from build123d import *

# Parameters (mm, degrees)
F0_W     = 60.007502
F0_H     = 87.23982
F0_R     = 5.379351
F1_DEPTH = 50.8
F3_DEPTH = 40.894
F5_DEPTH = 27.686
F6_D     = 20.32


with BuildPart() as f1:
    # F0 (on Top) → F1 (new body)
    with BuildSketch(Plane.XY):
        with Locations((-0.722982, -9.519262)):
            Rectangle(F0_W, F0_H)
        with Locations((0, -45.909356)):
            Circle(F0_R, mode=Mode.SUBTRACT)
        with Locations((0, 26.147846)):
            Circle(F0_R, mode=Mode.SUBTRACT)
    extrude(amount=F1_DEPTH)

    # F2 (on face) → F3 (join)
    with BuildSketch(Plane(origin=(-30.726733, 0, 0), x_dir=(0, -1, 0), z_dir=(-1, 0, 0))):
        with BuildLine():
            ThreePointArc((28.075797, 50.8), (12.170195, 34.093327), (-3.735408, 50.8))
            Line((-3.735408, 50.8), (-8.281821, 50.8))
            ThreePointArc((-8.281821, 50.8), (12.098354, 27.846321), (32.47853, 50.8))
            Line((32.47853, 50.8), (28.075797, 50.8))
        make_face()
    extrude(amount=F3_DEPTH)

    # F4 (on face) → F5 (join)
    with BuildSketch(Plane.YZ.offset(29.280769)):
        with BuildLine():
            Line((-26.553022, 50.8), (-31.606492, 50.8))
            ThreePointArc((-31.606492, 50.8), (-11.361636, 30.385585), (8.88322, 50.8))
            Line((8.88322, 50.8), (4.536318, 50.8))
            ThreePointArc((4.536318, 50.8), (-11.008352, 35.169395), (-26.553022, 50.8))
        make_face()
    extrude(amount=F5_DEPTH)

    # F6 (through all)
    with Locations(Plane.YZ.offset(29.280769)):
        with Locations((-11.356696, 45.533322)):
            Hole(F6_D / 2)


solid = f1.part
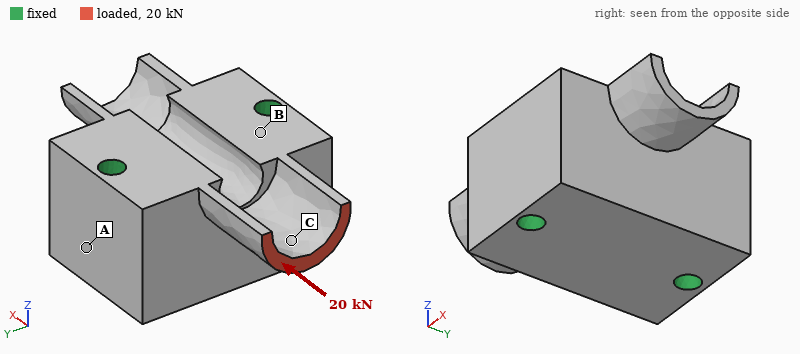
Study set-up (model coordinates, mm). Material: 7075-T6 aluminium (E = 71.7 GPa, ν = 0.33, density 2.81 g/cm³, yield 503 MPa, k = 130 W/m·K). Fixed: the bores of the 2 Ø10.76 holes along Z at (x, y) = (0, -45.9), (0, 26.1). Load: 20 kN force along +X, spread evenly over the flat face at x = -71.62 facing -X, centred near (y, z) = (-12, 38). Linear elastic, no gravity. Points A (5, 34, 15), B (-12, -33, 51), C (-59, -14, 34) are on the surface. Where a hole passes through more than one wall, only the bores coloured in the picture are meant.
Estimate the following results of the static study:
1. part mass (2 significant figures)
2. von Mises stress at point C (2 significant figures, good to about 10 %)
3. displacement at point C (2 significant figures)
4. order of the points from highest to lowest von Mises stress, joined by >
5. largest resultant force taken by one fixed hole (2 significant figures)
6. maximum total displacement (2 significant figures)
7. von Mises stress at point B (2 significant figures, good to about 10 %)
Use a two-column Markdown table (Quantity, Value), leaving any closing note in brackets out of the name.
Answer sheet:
| Quantity | Value |
|---|---|
| part mass | 740 g |
| von Mises stress at point C | 59 MPa |
| displacement at point C | 35 µm |
| order of the points from highest to lowest von Mises stress, joined by > | C > B > A |
| largest resultant force taken by one fixed hole | 11 kN |
| maximum total displacement | 49 µm |
| von Mises stress at point B | 21 MPa |
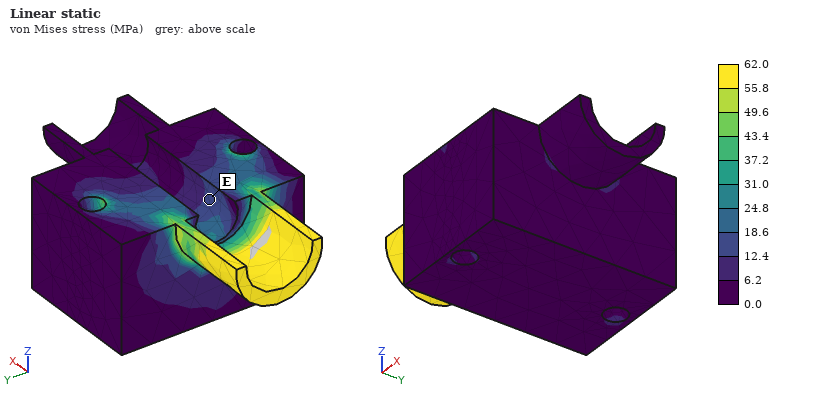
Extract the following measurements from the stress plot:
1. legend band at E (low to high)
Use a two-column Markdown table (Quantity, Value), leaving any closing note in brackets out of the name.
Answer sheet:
| Quantity | Value |
|---|---|
| legend band at E | 12.4 to 18.6 MPa |
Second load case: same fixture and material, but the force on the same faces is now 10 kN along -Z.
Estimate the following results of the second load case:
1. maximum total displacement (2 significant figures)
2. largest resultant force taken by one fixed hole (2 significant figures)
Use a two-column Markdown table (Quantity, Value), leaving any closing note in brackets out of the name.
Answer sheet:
| Quantity | Value |
|---|---|
| maximum total displacement | 0.55 mm |
| largest resultant force taken by one fixed hole | 5.3 kN |
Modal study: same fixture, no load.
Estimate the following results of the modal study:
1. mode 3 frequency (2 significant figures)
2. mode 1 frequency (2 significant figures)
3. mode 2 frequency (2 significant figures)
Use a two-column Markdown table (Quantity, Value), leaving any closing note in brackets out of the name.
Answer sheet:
| Quantity | Value |
|---|---|
| mode 3 frequency | 7800 Hz |
| mode 1 frequency | 5100 Hz |
| mode 2 frequency | 6400 Hz |
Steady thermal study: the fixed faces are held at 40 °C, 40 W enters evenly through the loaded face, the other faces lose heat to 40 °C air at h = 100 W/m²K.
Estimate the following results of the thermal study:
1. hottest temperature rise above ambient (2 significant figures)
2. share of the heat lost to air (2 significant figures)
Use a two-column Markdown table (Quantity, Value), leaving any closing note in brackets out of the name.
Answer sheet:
| Quantity | Value |
|---|---|
| hottest temperature rise above ambient | 36 K |
| share of the heat lost to air | 31 % |
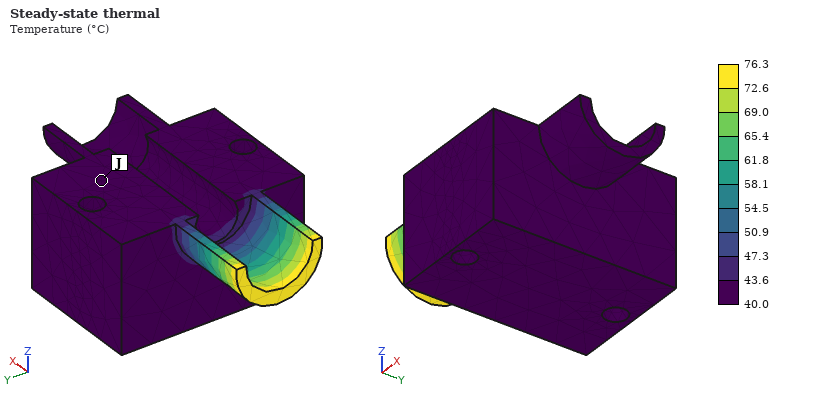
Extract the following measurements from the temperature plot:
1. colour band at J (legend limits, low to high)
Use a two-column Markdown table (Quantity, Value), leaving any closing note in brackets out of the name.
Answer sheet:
| Quantity | Value |
|---|---|
| colour band at J | 40.0 to 43.6 °C |
